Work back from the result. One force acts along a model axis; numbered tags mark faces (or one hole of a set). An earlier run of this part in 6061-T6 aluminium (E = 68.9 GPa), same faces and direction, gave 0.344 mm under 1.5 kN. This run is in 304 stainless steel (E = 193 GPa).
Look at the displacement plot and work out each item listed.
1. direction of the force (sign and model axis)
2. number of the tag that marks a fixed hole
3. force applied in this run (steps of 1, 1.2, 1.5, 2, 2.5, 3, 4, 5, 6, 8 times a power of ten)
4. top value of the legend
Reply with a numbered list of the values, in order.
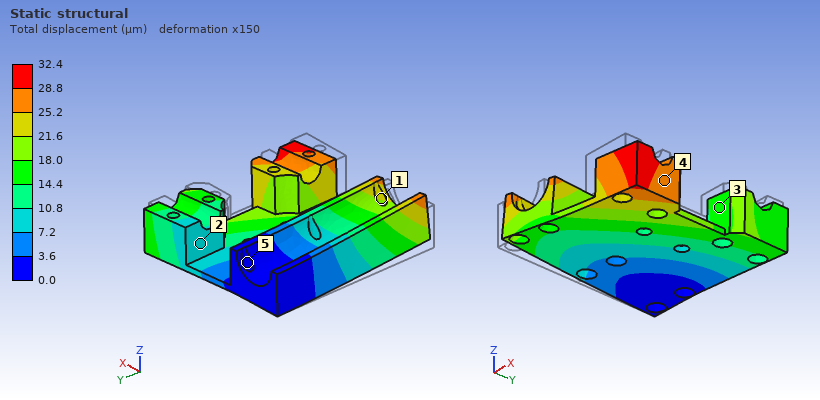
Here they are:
1. +X
2. 5
3. 400 N
4. 32.4 µm
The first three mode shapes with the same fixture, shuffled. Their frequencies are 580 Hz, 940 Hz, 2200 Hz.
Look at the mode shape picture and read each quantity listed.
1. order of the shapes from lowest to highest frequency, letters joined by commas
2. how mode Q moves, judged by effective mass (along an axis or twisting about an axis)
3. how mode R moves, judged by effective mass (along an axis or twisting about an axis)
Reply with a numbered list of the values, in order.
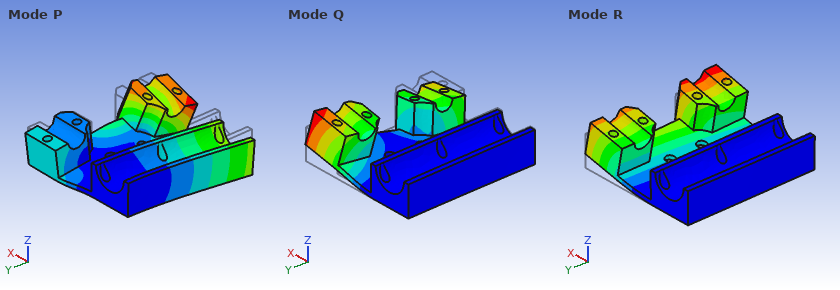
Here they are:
1. R, Q, P
2. twisting about X
3. along Z
